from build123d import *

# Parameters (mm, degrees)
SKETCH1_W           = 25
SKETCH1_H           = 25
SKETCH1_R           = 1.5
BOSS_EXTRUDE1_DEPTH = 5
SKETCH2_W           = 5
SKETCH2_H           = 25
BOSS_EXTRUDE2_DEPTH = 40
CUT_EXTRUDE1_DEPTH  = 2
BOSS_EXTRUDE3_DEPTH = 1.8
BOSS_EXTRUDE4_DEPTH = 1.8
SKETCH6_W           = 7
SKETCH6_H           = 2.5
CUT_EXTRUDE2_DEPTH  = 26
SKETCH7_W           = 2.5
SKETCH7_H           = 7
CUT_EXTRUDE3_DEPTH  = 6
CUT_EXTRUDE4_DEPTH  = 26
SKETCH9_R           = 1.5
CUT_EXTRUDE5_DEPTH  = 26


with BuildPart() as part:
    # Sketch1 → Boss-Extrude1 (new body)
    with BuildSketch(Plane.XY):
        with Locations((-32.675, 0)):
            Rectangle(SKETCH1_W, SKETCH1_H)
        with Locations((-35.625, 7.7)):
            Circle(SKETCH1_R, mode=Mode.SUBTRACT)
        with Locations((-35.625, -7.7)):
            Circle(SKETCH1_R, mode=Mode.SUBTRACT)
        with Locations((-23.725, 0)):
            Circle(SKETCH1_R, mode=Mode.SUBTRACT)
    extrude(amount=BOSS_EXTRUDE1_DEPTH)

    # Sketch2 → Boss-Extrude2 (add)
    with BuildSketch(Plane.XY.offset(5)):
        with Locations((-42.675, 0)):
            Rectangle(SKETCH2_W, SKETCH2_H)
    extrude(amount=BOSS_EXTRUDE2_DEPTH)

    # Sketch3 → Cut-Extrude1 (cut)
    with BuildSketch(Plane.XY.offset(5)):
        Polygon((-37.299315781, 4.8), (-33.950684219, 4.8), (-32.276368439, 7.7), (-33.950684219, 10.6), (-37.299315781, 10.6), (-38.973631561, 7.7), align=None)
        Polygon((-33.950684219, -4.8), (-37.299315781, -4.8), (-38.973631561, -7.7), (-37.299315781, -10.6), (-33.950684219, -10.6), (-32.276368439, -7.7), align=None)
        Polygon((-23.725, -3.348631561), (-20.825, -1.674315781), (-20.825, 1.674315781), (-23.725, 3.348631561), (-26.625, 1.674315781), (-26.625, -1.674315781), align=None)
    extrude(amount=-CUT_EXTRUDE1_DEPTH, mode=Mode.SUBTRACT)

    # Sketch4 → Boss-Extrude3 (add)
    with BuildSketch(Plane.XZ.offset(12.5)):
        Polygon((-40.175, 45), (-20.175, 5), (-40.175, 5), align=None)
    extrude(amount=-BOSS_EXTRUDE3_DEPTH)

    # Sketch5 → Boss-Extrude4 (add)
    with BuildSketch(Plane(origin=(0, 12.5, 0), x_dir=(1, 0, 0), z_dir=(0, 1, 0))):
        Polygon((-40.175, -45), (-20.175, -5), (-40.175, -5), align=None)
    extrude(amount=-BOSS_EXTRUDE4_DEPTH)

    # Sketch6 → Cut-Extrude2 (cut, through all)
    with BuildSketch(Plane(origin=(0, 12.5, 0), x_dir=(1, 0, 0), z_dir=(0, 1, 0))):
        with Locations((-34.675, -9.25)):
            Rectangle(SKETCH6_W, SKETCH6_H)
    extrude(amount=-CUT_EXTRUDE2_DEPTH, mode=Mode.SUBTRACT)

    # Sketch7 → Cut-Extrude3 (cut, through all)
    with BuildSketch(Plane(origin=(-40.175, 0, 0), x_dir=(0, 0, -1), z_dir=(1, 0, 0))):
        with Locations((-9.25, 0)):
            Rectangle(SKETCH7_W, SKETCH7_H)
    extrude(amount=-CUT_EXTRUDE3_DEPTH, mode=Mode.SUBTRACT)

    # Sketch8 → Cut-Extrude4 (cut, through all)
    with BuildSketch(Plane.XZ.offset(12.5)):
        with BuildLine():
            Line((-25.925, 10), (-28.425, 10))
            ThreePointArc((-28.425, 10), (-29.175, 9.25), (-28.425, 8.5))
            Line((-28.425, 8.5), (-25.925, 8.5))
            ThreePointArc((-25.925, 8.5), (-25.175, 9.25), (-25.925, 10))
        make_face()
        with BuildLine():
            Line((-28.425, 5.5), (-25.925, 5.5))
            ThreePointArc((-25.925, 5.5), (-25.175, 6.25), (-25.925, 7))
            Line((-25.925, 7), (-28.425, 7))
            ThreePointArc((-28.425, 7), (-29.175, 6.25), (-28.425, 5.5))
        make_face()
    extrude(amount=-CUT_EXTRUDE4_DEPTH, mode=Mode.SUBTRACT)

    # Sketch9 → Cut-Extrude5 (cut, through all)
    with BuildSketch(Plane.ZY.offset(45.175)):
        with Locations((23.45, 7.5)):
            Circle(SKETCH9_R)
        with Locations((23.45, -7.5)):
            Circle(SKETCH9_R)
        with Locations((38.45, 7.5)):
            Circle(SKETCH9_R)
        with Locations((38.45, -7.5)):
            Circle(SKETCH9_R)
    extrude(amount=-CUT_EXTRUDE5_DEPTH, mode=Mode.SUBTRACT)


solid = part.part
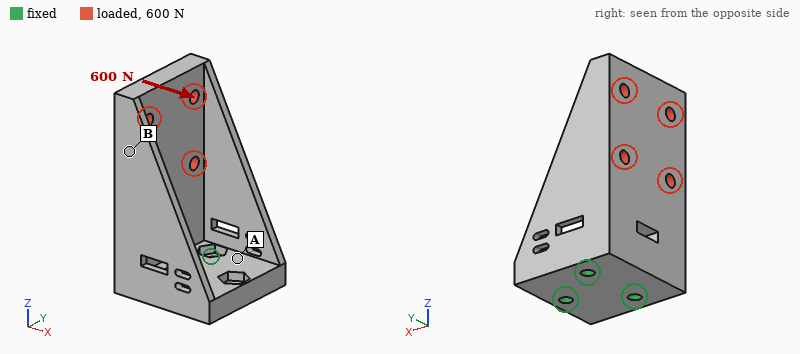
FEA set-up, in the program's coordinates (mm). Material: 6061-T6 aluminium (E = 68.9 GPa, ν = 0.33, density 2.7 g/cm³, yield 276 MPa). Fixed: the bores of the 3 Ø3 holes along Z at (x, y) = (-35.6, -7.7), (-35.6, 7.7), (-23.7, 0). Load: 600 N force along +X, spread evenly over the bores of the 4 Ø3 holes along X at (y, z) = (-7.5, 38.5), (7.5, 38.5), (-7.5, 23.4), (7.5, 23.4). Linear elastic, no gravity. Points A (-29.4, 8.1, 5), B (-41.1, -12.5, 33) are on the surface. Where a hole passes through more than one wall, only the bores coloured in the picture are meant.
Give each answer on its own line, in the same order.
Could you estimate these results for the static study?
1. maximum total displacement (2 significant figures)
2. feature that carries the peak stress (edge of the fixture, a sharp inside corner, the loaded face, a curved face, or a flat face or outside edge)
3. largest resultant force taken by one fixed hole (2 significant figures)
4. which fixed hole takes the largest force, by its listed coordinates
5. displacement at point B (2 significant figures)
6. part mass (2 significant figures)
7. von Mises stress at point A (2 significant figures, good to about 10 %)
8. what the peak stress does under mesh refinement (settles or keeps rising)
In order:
0.16 mm
edge of the fixture
1.0 kN
(-23.7, 0)
0.10 mm
24 g
56 MPa
keeps rising
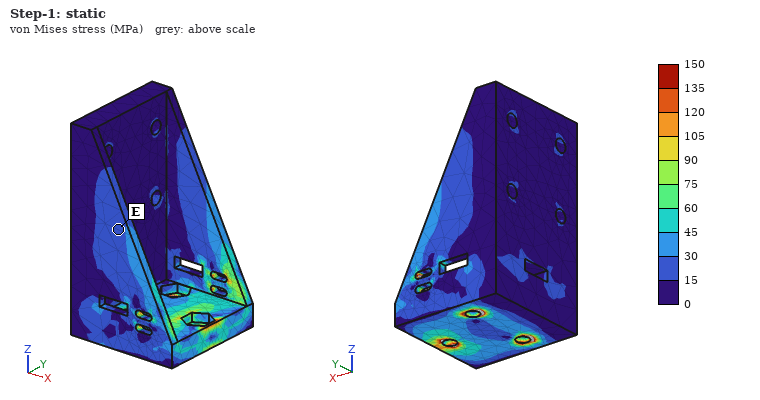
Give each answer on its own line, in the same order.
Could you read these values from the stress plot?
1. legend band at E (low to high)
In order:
15 to 30 MPa
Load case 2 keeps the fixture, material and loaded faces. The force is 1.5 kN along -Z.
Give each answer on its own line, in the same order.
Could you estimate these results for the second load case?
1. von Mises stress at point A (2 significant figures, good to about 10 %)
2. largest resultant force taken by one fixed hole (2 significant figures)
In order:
25 MPa
990 N
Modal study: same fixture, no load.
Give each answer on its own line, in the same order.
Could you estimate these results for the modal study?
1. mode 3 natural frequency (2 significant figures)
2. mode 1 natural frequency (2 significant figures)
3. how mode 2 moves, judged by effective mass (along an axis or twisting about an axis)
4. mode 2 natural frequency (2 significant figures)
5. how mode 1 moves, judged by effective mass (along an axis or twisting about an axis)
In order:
9200 Hz
3500 Hz
along Y
4600 Hz
along X
